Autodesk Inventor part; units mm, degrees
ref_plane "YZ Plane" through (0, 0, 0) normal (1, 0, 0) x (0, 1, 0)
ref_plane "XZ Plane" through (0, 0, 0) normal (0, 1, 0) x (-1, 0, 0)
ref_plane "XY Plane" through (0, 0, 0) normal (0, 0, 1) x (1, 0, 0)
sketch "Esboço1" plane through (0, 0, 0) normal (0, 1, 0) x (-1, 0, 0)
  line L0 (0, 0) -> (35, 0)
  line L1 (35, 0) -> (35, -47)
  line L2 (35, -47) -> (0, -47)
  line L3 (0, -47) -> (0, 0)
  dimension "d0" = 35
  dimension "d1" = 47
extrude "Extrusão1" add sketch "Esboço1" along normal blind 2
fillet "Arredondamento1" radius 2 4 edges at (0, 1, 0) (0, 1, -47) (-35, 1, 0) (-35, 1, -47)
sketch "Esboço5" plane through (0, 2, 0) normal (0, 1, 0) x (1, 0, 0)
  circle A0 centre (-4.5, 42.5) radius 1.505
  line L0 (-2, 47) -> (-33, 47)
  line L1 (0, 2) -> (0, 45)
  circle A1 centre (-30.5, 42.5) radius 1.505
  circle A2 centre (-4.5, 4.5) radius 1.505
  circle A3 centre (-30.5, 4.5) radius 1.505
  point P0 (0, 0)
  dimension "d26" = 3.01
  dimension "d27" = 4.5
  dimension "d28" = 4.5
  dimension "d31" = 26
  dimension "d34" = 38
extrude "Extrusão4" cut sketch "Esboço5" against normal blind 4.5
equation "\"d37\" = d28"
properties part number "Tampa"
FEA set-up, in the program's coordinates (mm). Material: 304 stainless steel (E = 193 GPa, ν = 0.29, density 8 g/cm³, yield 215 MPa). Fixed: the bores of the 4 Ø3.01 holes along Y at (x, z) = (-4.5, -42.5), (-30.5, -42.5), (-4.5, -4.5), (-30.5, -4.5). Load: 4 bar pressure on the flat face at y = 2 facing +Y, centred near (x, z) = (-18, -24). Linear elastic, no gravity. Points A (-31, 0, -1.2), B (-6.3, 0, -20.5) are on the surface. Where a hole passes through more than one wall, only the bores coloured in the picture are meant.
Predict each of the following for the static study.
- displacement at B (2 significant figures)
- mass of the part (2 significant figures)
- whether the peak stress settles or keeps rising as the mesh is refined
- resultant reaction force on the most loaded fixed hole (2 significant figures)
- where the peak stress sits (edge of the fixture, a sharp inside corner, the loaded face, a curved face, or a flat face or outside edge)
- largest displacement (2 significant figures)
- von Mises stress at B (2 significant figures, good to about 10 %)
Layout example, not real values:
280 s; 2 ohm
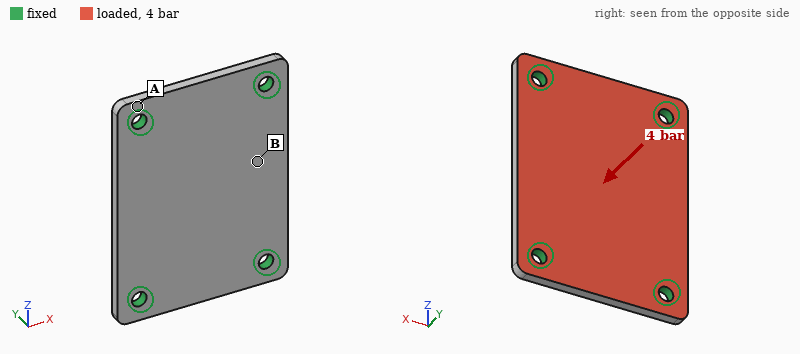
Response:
18 µm; 26 g; keeps rising; 160 N; edge of the fixture; 22 µm; 34 MPa
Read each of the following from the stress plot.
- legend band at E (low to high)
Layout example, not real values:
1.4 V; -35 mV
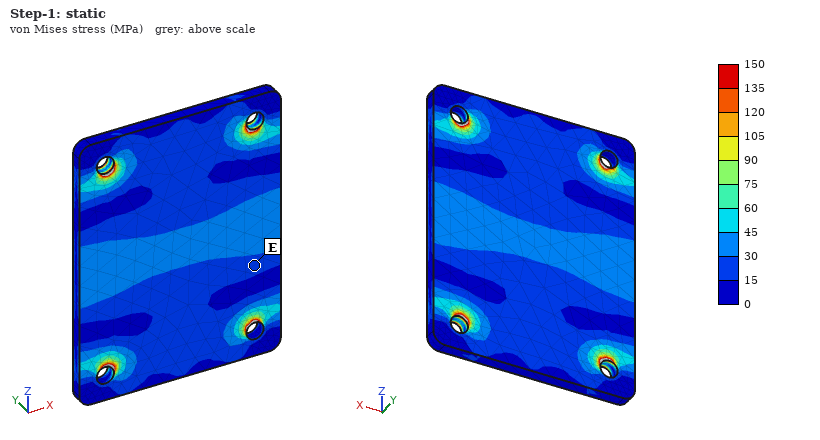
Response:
15 to 30 MPa
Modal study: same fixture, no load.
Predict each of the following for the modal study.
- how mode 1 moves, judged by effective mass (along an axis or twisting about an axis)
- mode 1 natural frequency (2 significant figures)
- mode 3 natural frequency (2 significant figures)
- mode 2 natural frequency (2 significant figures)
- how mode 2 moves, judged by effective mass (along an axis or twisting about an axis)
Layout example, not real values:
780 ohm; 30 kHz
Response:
along Y; 6300 Hz; 13 kHz; 8900 Hz; twisting about Z
